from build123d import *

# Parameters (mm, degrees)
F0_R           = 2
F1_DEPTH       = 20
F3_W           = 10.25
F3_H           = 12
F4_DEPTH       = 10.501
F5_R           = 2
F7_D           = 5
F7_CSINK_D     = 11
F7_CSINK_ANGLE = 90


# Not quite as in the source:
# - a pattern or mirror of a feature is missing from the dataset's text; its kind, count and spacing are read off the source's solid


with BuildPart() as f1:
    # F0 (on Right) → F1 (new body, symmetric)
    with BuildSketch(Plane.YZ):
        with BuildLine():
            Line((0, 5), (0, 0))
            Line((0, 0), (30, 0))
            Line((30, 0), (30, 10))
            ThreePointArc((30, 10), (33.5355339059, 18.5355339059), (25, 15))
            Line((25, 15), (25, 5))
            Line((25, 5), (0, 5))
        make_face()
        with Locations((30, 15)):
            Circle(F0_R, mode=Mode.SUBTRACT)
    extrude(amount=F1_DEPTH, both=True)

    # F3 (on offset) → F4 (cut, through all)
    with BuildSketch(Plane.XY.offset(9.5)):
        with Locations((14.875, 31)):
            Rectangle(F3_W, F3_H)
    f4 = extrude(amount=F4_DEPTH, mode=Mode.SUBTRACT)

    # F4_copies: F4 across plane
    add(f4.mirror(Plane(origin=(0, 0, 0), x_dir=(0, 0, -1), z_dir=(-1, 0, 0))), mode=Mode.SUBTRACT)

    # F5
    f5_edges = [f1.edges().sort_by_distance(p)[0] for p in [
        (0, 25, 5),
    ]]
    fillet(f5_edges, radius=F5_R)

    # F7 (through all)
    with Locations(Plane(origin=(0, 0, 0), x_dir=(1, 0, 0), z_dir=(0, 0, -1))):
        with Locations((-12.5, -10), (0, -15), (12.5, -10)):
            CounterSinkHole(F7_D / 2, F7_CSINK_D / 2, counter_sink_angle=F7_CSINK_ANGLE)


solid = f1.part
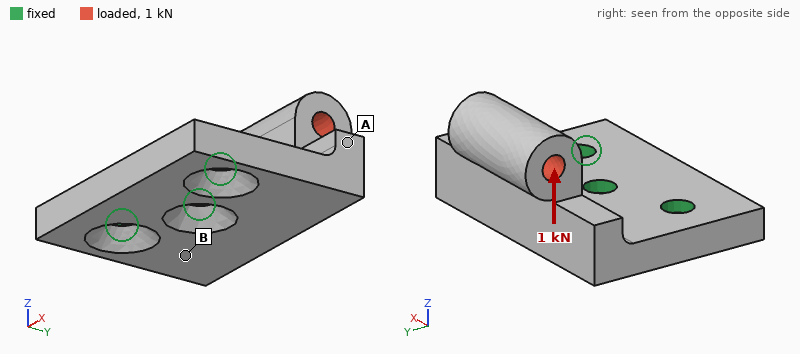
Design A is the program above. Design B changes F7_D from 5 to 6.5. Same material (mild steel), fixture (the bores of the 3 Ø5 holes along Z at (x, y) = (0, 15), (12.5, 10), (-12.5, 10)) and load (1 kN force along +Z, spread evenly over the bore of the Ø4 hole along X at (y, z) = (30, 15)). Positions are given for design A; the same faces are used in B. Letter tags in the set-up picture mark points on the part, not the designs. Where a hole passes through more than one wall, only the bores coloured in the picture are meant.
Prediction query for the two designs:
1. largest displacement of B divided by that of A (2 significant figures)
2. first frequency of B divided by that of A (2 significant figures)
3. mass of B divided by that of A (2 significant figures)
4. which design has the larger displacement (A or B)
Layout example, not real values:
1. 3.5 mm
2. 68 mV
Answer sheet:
1. 0.73
2. 1.2
3. 0.99
4. A
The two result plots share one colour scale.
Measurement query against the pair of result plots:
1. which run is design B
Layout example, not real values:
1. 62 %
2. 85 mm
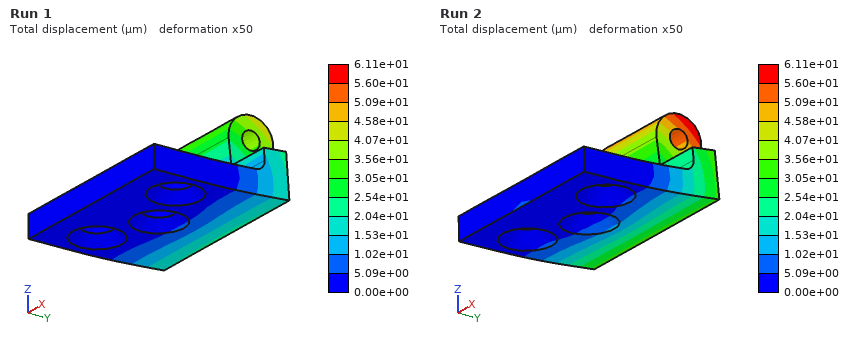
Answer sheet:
1. Run 1
